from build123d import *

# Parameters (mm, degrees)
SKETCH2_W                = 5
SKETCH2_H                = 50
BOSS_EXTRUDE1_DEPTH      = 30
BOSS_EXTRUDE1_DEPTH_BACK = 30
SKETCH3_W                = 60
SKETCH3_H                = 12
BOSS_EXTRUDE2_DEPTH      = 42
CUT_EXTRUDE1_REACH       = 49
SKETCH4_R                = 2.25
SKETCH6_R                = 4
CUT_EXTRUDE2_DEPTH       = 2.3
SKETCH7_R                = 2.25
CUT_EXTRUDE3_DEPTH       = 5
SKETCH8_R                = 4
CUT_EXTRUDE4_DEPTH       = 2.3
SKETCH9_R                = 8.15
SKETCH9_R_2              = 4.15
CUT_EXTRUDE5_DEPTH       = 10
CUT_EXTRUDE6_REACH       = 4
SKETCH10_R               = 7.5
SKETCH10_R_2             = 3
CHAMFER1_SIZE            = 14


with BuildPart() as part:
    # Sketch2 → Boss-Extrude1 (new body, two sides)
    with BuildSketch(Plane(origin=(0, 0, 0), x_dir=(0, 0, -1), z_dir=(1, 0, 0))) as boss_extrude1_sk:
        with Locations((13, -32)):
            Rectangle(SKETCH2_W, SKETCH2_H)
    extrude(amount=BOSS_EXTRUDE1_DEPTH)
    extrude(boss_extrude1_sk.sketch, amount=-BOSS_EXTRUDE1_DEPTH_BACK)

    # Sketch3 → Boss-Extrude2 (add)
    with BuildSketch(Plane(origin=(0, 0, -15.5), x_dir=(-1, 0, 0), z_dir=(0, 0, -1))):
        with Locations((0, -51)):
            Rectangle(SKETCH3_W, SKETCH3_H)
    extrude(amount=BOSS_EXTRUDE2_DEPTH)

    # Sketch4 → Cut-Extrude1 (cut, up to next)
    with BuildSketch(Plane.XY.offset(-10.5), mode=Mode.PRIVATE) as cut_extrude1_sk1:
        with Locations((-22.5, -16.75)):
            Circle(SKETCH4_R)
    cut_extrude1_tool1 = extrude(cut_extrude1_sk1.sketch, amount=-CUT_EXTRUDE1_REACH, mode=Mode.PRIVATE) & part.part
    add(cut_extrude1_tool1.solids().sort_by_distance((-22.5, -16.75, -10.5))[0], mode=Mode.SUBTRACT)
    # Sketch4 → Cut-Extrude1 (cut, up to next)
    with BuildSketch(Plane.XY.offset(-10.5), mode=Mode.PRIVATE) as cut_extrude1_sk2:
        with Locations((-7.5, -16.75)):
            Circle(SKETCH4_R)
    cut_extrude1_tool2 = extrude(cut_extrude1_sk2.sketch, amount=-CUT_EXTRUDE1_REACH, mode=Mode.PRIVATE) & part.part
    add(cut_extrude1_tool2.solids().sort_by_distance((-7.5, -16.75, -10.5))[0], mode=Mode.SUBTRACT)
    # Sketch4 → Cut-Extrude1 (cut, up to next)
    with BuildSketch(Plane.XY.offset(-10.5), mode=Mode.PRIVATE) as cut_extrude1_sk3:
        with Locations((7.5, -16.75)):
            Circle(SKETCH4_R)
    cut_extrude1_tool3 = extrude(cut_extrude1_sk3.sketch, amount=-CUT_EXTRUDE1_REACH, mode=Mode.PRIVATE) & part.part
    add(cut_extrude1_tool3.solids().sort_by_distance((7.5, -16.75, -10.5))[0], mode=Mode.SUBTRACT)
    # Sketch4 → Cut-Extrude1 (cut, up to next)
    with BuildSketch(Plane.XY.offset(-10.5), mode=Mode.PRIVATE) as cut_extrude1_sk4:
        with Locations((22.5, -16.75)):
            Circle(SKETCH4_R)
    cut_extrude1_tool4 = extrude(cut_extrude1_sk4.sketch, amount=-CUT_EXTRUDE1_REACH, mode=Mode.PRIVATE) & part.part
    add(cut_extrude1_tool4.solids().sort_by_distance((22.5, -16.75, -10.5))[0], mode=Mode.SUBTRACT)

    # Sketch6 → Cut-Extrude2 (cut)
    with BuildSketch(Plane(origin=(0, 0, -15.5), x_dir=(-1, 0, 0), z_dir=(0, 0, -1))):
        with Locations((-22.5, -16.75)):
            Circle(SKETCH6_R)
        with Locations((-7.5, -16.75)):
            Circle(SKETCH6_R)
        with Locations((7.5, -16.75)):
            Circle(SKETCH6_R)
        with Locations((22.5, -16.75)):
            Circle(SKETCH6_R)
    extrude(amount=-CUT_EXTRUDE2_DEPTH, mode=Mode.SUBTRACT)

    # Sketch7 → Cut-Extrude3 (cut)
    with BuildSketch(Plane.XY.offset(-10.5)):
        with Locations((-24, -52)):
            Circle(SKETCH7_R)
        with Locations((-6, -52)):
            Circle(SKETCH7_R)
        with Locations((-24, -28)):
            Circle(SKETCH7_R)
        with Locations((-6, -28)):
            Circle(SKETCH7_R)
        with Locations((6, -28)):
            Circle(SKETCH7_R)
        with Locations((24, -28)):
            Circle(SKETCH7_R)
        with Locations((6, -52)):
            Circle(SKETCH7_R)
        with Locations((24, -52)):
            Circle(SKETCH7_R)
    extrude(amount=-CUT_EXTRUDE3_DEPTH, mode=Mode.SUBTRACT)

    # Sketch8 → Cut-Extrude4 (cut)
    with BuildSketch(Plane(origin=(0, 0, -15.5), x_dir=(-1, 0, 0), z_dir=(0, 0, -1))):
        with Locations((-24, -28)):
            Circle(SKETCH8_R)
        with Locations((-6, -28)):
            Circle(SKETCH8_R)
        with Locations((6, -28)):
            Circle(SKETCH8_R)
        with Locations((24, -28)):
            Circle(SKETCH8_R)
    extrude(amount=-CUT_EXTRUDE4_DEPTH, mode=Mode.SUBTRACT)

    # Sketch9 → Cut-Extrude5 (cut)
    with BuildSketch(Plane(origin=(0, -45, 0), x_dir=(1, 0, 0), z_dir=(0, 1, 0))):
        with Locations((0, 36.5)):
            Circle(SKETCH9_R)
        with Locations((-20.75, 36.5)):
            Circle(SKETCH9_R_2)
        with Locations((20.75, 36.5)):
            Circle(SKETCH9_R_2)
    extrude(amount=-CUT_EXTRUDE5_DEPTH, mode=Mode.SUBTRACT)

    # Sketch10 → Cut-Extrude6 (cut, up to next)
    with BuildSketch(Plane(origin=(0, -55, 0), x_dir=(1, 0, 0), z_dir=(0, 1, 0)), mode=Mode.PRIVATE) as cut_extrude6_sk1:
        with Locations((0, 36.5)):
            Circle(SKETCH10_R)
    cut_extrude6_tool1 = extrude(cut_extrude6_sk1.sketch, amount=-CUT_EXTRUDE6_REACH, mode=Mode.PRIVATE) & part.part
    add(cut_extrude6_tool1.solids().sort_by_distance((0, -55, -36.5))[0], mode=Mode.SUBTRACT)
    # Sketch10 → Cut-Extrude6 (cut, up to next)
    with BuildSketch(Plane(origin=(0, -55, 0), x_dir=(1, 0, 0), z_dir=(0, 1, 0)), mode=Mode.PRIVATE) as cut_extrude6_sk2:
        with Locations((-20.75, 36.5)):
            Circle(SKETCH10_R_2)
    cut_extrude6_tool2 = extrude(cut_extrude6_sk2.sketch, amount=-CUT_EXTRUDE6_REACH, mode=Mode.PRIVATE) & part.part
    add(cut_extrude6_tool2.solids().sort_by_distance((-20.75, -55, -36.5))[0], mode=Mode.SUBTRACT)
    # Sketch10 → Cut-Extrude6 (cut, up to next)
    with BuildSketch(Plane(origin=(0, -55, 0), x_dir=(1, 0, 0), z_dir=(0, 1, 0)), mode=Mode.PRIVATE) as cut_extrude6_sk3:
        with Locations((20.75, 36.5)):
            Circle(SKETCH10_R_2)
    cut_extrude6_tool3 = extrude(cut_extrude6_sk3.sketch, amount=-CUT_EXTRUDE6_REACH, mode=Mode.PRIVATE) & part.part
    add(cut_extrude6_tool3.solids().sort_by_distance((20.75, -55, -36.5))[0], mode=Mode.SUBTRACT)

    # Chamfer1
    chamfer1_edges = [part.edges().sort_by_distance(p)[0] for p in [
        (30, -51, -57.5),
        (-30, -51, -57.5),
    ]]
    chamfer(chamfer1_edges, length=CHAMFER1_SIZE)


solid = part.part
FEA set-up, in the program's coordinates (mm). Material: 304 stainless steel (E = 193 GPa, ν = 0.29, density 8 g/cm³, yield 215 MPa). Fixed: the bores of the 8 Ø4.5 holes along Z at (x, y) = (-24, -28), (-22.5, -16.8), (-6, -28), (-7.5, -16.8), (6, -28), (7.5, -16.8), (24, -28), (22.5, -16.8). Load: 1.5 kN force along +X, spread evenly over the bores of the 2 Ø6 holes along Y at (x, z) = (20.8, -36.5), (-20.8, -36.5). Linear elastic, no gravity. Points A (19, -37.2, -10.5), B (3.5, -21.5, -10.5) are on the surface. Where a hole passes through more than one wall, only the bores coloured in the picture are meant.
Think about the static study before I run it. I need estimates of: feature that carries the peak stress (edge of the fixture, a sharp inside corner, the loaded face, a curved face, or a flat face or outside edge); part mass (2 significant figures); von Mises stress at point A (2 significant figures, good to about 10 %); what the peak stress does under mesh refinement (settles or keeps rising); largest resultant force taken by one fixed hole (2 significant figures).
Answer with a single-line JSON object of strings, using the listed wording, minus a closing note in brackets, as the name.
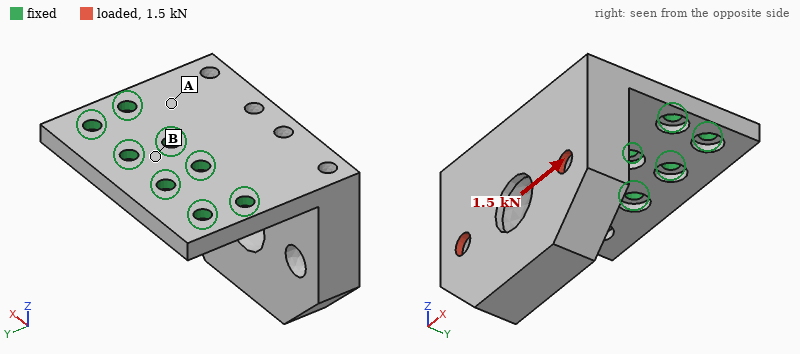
{"feature that carries the peak stress": "edge of the fixture", "part mass": "300 g", "von Mises stress at point A": "24 MPa", "what the peak stress does under mesh refinement": "keeps rising", "largest resultant force taken by one fixed hole": "1.3 kN"}
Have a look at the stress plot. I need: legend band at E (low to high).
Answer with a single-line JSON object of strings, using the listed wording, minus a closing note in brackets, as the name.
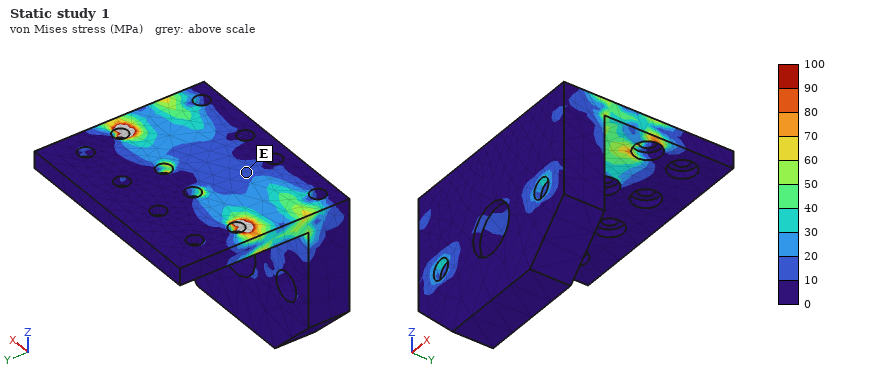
{"legend band at E": "10 to 20 MPa"}
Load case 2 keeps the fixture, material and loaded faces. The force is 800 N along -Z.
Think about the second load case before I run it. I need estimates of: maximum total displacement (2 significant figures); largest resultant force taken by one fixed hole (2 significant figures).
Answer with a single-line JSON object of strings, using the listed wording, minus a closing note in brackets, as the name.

{"maximum total displacement": "0.15 mm", "largest resultant force taken by one fixed hole": "590 N"}
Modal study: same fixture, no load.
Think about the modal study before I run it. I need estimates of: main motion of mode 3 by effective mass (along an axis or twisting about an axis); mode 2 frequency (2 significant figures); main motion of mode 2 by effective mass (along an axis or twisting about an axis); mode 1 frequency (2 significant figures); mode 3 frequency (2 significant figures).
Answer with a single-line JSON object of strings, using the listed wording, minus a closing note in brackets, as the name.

{"main motion of mode 3 by effective mass": "along Z", "mode 2 frequency": "2300 Hz", "main motion of mode 2 by effective mass": "along X", "mode 1 frequency": "870 Hz", "mode 3 frequency": "4200 Hz"}
